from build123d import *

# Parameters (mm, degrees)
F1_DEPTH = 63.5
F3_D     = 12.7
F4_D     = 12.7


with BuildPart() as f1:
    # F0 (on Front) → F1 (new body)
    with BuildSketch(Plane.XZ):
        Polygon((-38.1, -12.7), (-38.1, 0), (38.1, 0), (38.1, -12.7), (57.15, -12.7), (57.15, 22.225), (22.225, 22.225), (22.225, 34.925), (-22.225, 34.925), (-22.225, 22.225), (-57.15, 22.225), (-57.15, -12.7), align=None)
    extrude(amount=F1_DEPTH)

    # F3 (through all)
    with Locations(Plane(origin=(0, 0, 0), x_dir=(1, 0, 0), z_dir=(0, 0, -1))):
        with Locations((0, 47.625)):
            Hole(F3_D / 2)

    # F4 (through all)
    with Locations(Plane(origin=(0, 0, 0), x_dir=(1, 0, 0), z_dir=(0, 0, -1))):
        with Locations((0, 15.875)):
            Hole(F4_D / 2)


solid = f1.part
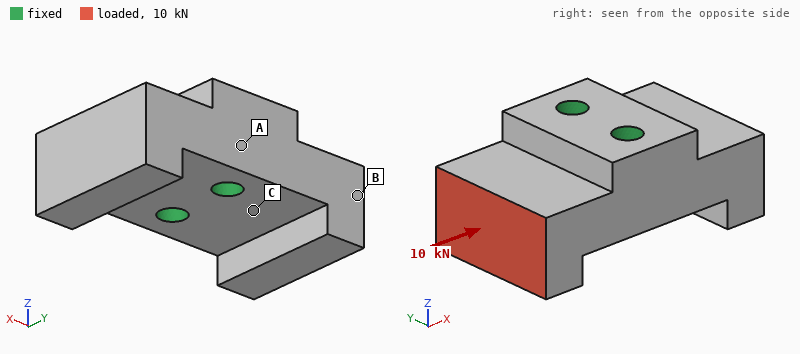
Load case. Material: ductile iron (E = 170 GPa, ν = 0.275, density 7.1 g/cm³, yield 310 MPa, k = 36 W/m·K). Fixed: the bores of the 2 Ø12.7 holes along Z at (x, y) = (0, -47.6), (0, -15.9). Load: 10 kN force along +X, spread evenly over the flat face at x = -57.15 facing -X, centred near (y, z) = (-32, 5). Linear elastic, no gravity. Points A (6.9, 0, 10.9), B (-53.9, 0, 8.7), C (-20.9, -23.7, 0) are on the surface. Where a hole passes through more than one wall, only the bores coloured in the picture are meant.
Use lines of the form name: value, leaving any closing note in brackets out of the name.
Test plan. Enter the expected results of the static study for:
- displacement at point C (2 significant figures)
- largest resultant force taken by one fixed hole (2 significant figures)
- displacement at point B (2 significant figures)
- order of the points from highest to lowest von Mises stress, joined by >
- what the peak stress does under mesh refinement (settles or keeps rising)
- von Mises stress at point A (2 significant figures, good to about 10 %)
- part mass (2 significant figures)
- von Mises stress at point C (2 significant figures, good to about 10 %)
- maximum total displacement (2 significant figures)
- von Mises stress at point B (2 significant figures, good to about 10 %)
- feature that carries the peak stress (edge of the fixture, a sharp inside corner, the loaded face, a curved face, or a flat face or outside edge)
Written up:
displacement at point C: 2.1 µm
largest resultant force taken by one fixed hole: 5.0 kN
displacement at point B: 7.2 µm
order of the points from highest to lowest von Mises stress, joined by >: C > B > A
what the peak stress does under mesh refinement: keeps rising
von Mises stress at point A: 2.9 MPa
part mass: 1.6 kg
von Mises stress at point C: 18 MPa
maximum total displacement: 12 µm
von Mises stress at point B: 7.1 MPa
feature that carries the peak stress: edge of the fixture
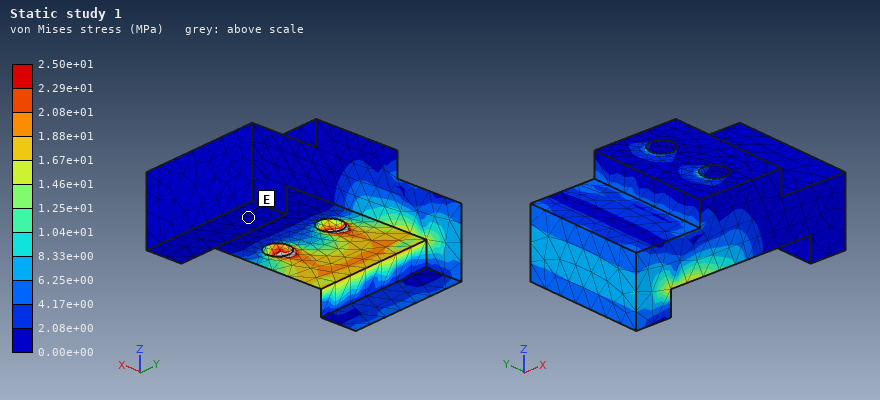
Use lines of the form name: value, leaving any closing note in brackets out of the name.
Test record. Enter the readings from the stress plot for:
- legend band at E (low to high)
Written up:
legend band at E: 0.00e+00 to 2.08e+00 MPa
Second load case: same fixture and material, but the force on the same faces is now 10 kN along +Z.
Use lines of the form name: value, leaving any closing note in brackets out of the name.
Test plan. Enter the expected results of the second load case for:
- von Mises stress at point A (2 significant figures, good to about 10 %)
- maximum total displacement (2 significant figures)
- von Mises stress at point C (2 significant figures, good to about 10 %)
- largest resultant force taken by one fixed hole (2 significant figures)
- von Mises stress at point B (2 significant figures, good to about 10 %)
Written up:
von Mises stress at point A: 7.0 MPa
maximum total displacement: 47 µm
von Mises stress at point C: 55 MPa
largest resultant force taken by one fixed hole: 5.0 kN
von Mises stress at point B: 17 MPa
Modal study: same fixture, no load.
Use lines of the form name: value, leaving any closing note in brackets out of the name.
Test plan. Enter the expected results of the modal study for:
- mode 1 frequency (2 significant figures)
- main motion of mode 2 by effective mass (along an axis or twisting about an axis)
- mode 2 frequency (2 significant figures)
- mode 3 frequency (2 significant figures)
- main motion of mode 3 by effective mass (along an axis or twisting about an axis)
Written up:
mode 1 frequency: 5400 Hz
main motion of mode 2 by effective mass: along Z
mode 2 frequency: 5600 Hz
mode 3 frequency: 7900 Hz
main motion of mode 3 by effective mass: twisting about Z
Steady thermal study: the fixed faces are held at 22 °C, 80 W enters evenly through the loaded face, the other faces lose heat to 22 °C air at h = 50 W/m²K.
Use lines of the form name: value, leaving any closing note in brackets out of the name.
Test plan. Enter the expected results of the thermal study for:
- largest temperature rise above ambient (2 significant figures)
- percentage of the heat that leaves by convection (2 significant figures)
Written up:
largest temperature rise above ambient: 64 K
percentage of the heat that leaves by convection: 22 %
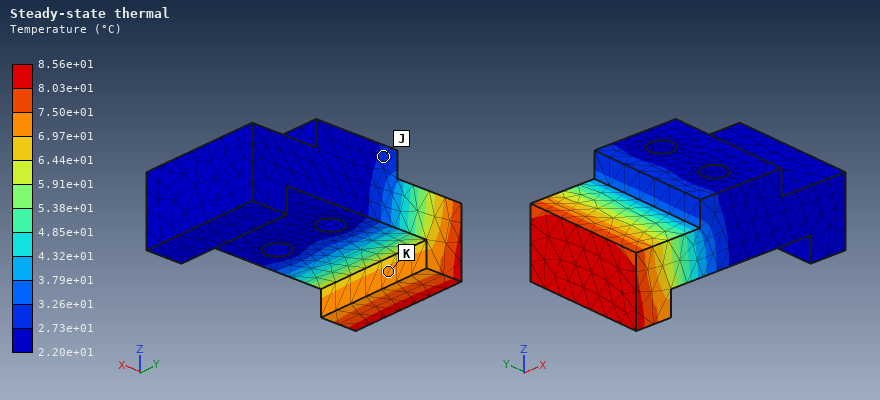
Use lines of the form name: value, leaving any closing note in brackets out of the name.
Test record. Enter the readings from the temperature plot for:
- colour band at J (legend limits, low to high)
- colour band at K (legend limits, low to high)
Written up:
colour band at J: 2.73e+01 to 3.26e+01 °C
colour band at K: 6.97e+01 to 7.50e+01 °C
